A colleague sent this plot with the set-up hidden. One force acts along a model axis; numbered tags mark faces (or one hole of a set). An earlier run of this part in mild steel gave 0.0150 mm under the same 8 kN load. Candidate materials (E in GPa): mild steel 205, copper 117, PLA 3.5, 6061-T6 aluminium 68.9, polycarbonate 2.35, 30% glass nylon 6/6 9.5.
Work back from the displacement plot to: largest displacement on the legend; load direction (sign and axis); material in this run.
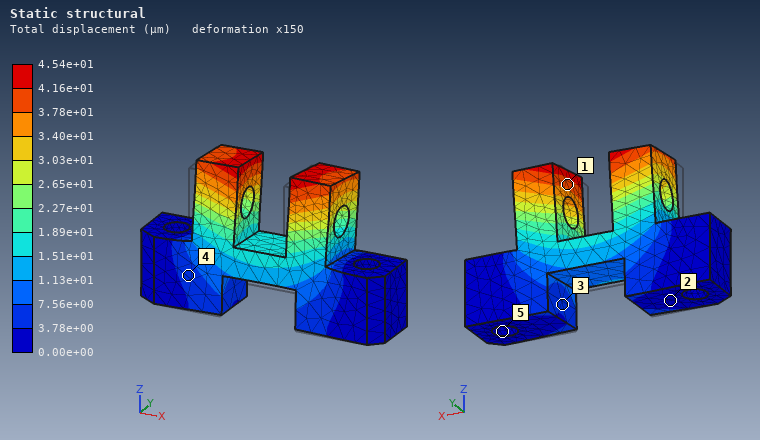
4.54e+01 µm
+Y
6061-T6 aluminium
